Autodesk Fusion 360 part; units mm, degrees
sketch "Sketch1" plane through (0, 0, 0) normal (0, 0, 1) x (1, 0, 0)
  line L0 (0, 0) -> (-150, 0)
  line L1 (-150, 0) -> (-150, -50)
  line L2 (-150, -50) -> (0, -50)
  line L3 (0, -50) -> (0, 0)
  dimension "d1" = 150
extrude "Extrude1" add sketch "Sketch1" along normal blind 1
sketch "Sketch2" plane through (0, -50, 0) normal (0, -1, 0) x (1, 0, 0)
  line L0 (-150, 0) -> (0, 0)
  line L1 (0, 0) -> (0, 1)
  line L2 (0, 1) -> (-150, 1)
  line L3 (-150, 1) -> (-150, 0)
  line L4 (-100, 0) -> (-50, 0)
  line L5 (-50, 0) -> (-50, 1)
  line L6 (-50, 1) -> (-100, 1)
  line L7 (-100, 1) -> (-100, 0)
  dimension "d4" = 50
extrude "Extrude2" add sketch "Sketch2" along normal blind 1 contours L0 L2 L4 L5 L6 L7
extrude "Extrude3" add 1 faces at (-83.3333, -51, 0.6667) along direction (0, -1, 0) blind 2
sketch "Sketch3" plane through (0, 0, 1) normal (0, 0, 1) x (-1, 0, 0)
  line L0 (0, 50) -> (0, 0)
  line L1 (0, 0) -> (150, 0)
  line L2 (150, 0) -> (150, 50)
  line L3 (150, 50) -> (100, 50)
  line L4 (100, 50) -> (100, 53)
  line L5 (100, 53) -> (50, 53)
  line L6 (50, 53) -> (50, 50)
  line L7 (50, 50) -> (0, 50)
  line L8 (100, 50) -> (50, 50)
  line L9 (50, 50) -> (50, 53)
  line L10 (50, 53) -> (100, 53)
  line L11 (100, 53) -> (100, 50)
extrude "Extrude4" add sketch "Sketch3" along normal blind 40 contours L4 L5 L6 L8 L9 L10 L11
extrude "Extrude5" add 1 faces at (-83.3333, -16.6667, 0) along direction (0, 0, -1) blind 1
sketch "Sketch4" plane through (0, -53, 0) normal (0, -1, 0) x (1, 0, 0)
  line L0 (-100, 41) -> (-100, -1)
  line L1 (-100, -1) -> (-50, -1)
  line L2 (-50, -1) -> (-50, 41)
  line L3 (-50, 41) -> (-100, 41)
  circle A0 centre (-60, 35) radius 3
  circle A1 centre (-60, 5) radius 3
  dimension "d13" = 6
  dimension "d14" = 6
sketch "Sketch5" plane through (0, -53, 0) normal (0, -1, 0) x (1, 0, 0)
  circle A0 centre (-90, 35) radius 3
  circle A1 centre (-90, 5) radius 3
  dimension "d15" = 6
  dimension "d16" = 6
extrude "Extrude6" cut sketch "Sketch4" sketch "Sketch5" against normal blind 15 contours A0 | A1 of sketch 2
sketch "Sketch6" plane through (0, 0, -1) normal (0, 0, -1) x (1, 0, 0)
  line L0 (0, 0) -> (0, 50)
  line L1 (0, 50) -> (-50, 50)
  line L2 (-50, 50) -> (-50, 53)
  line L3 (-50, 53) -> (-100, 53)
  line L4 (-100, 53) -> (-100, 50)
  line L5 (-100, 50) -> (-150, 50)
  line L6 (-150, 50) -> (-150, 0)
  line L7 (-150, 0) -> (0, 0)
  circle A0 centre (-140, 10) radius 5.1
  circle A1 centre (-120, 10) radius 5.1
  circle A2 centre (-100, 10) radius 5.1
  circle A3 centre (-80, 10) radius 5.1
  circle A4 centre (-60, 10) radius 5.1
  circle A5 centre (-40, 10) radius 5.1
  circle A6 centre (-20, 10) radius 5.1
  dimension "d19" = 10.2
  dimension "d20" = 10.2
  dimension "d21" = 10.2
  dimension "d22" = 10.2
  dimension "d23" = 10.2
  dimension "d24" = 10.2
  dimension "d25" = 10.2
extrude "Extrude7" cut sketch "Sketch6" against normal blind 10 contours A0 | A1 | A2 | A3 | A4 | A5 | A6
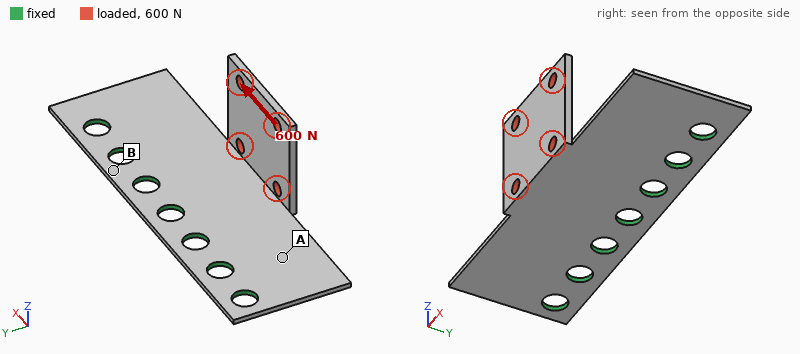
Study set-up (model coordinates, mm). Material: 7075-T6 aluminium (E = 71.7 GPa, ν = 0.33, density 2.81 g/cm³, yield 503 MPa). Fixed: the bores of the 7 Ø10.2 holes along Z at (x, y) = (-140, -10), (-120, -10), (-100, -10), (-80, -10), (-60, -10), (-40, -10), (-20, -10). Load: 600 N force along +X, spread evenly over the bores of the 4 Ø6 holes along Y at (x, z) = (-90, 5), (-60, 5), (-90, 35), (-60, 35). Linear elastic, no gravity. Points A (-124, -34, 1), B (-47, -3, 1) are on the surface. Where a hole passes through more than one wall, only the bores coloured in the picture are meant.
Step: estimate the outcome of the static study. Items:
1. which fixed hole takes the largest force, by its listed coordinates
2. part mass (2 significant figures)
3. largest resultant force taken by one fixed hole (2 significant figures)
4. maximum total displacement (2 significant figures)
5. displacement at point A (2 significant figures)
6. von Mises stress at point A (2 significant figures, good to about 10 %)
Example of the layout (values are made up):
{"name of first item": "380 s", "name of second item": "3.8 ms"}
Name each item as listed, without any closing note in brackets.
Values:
{"which fixed hole takes the largest force, by its listed coordinates": "(-20, -10)", "part mass": "56 g", "largest resultant force taken by one fixed hole": "170 N", "maximum total displacement": "1.2 mm", "displacement at point A": "0.21 mm", "von Mises stress at point A": "37 MPa"}
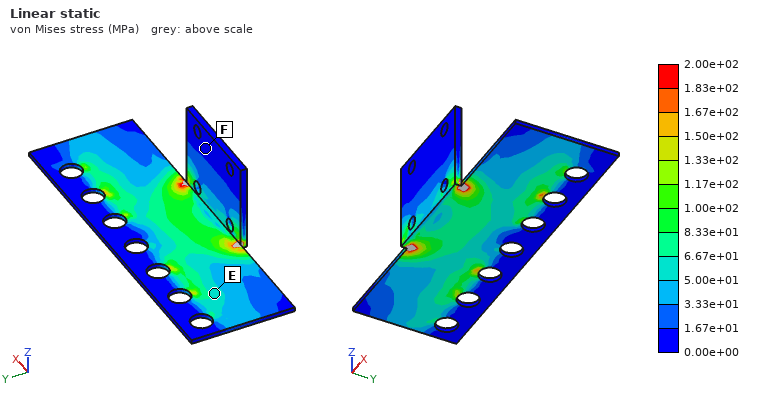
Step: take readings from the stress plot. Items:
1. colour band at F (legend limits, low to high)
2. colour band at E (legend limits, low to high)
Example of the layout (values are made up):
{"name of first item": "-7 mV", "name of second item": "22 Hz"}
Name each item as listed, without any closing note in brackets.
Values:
{"colour band at F": "0.00e+00 to 1.67e+01 MPa", "colour band at E": "5.00e+01 to 6.67e+01 MPa"}
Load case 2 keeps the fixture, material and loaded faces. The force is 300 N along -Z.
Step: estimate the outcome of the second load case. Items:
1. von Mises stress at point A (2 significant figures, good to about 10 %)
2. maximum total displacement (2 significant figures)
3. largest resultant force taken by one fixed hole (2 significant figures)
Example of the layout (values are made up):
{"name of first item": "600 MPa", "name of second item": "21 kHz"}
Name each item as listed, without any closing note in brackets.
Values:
{"von Mises stress at point A": "53 MPa", "maximum total displacement": "1.8 mm", "largest resultant force taken by one fixed hole": "71 N"}
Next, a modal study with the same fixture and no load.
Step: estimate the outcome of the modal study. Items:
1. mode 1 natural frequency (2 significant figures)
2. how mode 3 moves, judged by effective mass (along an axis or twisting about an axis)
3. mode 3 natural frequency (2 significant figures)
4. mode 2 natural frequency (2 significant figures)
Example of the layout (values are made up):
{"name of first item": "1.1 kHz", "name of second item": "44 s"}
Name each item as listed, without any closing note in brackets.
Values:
{"mode 1 natural frequency": "450 Hz", "how mode 3 moves, judged by effective mass": "along Z", "mode 3 natural frequency": "1100 Hz", "mode 2 natural frequency": "890 Hz"}
